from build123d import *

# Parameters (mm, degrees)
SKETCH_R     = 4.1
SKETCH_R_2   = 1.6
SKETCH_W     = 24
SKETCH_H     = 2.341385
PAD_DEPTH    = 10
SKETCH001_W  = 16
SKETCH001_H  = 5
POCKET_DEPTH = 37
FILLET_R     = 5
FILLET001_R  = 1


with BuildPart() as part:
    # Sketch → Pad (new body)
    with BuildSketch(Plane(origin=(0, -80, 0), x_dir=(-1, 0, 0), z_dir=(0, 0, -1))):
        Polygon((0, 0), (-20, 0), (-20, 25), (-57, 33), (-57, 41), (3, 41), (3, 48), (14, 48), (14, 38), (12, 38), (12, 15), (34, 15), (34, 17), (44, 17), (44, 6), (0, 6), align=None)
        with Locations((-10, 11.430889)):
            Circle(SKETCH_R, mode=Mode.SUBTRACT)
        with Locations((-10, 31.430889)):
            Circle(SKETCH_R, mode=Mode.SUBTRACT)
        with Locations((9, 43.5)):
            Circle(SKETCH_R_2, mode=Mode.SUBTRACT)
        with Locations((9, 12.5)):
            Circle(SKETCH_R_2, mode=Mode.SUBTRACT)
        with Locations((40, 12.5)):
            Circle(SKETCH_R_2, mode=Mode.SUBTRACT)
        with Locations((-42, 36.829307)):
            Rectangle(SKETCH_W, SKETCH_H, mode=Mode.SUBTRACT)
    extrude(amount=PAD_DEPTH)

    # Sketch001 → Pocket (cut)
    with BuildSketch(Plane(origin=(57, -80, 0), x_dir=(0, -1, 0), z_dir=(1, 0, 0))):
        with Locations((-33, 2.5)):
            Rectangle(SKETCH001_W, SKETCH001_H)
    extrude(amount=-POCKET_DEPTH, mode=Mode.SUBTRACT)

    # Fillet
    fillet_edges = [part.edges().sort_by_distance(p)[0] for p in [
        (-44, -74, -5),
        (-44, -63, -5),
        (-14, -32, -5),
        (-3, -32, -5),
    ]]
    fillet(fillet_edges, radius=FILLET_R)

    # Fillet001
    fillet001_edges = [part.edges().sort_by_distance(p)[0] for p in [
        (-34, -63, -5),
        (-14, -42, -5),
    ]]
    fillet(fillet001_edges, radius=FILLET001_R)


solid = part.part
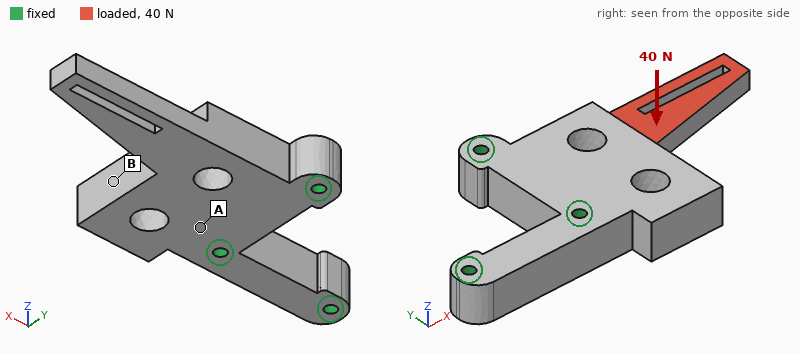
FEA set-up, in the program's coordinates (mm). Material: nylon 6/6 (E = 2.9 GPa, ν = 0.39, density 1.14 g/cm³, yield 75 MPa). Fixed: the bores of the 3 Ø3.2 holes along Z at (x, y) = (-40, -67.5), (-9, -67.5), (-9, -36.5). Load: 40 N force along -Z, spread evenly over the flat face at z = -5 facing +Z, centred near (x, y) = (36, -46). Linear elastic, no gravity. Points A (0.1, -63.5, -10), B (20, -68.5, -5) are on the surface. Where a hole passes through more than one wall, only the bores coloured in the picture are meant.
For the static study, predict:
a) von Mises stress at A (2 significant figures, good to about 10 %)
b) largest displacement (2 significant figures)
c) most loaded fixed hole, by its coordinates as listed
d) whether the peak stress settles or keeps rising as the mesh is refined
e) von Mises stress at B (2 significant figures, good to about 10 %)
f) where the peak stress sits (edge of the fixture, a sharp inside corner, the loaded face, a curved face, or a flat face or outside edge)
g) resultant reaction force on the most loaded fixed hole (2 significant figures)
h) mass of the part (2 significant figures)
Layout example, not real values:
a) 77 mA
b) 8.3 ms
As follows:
a) 3.1 MPa
b) 1.1 mm
c) (-9, -36.5)
d) keeps rising
e) 1.2 MPa
f) edge of the fixture
g) 28 N
h) 19 g
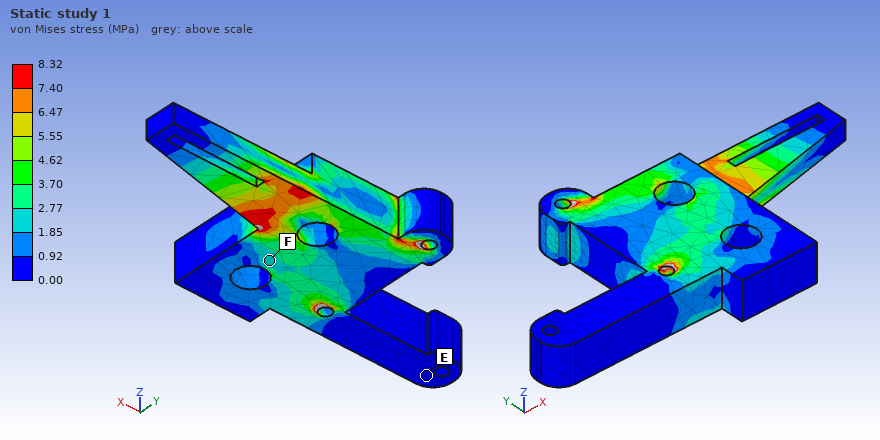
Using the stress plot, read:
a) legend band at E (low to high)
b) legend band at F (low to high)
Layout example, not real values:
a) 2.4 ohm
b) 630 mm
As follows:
a) 0.00 to 0.92 MPa
b) 1.85 to 2.77 MPa
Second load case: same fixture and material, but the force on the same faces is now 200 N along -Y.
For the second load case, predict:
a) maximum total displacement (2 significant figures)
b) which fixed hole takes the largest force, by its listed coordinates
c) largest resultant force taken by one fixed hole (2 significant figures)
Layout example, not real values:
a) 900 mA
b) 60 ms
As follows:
a) 1.00 mm
b) (-9, -36.5)
c) 310 N
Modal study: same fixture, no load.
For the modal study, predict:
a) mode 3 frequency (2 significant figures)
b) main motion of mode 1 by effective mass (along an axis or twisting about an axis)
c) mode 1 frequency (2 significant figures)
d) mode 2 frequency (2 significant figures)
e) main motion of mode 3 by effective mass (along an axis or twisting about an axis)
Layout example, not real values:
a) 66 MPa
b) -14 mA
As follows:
a) 2100 Hz
b) along Z
c) 820 Hz
d) 2000 Hz
e) along Z
